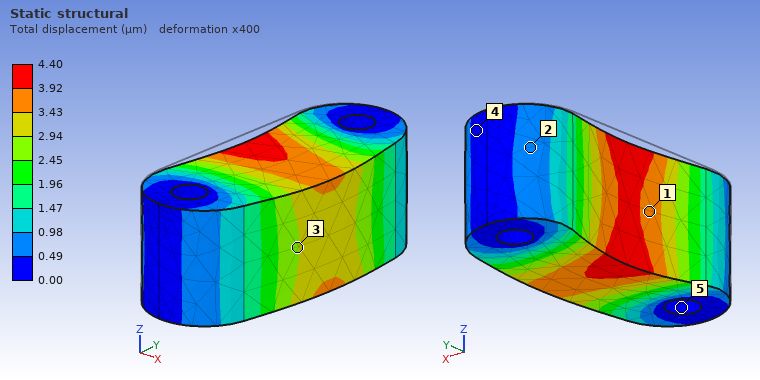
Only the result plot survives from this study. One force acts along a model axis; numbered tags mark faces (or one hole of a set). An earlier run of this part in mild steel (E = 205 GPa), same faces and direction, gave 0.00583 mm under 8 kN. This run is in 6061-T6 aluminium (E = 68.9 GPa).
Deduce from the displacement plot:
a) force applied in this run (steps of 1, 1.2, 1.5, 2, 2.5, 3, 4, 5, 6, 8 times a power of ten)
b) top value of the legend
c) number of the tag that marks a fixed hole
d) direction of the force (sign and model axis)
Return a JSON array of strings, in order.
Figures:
["2 kN", "4.40 µm", "5", "+X"]
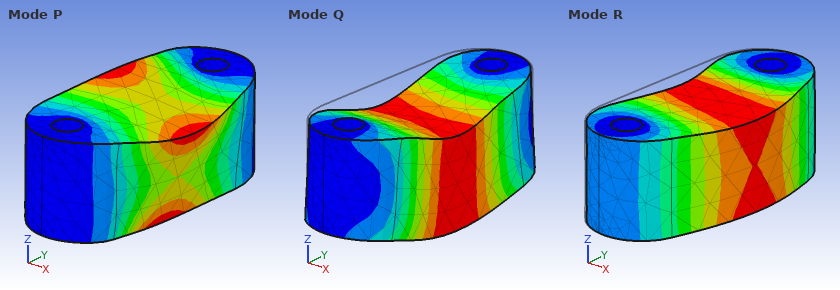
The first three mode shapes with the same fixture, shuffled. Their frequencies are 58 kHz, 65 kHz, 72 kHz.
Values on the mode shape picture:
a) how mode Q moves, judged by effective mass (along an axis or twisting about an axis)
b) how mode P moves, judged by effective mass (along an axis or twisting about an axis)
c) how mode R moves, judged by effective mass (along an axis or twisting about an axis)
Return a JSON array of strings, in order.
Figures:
["along Z", "twisting about Y", "along X"]
